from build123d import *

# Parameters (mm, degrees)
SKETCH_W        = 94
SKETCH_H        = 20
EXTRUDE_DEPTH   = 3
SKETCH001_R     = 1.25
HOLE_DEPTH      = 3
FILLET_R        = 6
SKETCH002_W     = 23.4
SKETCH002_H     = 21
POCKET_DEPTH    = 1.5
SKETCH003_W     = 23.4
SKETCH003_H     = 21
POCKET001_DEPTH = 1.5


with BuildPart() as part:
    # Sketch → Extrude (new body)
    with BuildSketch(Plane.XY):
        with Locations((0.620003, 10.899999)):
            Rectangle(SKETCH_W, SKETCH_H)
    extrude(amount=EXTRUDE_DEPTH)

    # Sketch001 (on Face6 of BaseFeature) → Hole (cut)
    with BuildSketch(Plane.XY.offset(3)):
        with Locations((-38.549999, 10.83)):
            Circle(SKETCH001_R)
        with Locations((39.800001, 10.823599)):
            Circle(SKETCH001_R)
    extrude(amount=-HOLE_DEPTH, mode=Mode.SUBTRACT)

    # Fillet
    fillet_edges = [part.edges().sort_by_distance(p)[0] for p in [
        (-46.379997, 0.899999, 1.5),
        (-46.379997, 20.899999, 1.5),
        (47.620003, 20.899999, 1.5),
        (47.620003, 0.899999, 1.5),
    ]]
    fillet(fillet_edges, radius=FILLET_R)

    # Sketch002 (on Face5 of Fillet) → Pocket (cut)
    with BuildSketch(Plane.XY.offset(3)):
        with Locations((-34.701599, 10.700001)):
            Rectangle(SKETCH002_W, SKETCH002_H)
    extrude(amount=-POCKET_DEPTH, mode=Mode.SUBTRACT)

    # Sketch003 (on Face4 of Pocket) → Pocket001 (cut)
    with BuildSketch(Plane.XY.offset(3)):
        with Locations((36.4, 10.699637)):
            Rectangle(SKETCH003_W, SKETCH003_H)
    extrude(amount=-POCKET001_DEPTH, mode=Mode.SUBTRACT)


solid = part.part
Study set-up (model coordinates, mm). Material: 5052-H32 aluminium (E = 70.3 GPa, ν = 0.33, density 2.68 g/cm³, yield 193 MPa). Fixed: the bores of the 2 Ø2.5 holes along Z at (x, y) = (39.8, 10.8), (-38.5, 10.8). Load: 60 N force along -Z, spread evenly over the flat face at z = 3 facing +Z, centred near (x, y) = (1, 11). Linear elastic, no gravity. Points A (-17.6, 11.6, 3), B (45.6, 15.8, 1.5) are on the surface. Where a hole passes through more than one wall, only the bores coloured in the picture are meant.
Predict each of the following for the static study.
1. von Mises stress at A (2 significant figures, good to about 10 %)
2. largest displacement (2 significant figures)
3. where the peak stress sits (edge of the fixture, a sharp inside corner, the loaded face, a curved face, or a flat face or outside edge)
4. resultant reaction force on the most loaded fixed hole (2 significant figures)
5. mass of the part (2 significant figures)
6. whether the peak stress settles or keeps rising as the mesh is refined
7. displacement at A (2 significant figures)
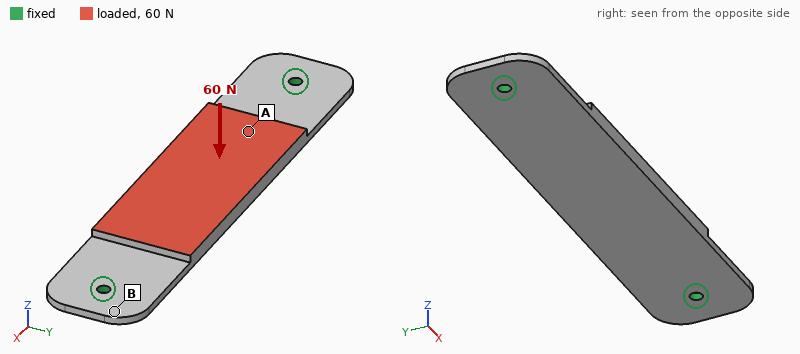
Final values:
10 MPa
84 µm
edge of the fixture
110 N
11 g
keeps rising
61 µm
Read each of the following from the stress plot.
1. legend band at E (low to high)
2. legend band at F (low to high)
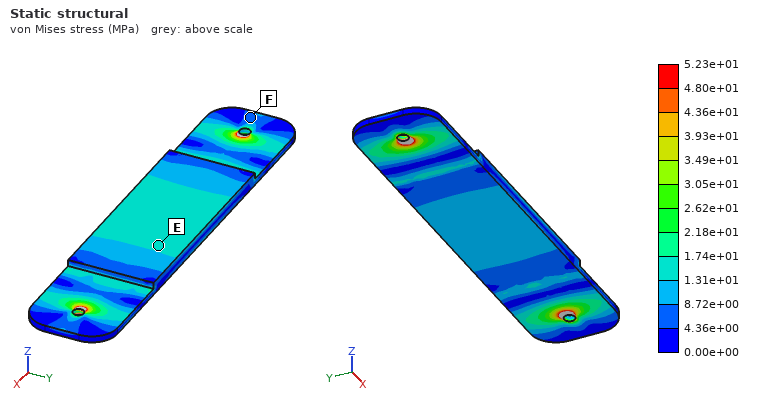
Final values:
1.31e+01 to 1.74e+01 MPa
4.36e+00 to 8.72e+00 MPa
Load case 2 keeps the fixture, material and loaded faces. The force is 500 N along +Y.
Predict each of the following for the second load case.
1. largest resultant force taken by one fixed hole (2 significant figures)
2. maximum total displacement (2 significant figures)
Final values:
250 N
0.16 mm
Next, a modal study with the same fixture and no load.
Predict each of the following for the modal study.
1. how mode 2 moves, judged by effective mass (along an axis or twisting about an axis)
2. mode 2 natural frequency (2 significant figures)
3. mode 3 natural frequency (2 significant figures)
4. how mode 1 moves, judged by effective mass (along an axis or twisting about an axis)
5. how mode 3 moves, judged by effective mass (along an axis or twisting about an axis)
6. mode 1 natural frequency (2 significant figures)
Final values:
twisting about X
2600 Hz
4200 Hz
along Z
twisting about Y
1600 Hz
